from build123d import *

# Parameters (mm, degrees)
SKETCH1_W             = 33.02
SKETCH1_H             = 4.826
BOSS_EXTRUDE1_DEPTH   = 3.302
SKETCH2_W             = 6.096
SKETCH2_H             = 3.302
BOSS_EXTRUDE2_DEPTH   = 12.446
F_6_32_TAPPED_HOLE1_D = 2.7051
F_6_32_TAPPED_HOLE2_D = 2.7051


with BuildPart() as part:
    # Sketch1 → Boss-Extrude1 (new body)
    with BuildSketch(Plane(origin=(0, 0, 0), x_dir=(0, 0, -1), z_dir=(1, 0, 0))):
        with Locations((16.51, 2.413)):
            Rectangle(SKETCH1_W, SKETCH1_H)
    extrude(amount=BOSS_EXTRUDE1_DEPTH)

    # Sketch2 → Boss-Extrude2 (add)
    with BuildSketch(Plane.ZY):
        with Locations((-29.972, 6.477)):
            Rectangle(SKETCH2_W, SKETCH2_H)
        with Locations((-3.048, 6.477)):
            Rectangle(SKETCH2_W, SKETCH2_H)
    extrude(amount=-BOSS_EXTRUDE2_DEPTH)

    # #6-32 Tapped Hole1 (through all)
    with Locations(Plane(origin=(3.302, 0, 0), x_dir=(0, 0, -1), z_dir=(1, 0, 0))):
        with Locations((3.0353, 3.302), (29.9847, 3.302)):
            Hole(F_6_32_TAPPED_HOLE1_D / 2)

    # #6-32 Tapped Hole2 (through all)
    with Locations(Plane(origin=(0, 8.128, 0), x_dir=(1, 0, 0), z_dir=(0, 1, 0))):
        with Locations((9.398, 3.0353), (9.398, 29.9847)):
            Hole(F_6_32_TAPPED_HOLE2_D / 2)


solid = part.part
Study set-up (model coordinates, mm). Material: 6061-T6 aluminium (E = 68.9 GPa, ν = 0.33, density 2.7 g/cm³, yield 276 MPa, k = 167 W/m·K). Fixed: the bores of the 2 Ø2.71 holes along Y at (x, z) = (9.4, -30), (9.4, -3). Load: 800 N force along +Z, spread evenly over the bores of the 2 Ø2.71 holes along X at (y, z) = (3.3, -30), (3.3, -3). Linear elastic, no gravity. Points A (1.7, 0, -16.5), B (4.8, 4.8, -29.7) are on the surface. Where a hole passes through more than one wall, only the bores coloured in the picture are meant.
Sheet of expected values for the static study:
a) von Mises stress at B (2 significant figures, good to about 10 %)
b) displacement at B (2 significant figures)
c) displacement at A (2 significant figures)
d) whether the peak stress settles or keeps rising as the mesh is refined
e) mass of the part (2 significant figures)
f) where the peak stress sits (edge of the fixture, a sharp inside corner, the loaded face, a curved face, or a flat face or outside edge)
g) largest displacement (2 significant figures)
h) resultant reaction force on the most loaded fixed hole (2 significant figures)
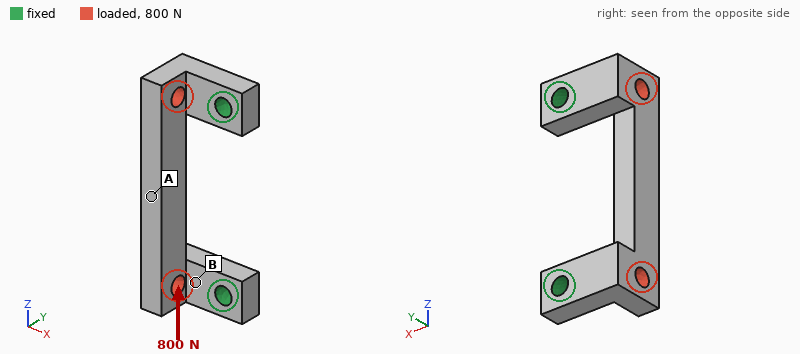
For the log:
92 MPa
12 µm
26 µm
keeps rising
2.6 g
a sharp inside corner
36 µm
410 N
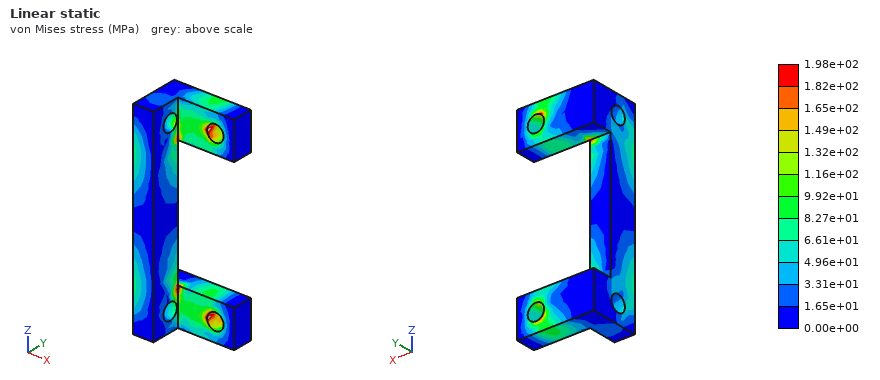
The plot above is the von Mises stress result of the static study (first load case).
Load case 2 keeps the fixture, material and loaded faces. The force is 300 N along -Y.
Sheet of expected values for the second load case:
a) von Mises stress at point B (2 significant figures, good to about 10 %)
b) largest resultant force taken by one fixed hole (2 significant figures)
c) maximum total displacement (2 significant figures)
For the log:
43 MPa
150 N
29 µm
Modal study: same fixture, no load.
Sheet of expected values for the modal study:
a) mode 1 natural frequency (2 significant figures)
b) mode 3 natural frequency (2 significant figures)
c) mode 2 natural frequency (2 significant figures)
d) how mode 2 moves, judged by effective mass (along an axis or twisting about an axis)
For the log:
11 kHz
21 kHz
19 kHz
along Z
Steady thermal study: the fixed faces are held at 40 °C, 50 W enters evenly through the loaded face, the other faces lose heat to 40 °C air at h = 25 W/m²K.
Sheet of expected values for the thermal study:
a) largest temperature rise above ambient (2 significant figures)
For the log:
74 K
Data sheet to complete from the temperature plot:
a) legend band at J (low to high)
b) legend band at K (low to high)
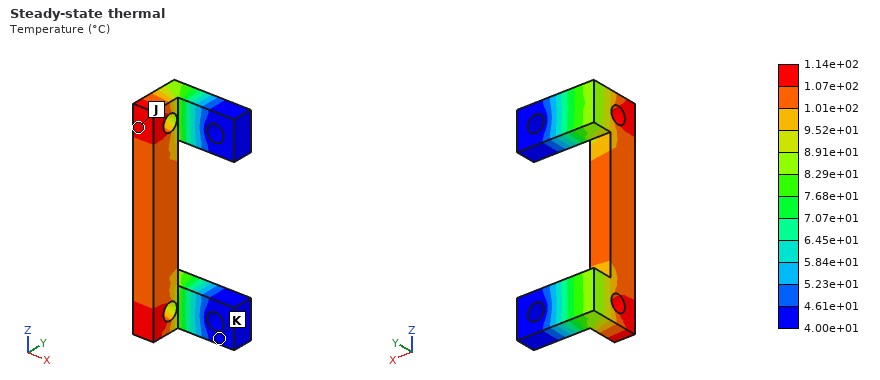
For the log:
1.07e+02 to 1.14e+02 °C
4.00e+01 to 4.61e+01 °C
